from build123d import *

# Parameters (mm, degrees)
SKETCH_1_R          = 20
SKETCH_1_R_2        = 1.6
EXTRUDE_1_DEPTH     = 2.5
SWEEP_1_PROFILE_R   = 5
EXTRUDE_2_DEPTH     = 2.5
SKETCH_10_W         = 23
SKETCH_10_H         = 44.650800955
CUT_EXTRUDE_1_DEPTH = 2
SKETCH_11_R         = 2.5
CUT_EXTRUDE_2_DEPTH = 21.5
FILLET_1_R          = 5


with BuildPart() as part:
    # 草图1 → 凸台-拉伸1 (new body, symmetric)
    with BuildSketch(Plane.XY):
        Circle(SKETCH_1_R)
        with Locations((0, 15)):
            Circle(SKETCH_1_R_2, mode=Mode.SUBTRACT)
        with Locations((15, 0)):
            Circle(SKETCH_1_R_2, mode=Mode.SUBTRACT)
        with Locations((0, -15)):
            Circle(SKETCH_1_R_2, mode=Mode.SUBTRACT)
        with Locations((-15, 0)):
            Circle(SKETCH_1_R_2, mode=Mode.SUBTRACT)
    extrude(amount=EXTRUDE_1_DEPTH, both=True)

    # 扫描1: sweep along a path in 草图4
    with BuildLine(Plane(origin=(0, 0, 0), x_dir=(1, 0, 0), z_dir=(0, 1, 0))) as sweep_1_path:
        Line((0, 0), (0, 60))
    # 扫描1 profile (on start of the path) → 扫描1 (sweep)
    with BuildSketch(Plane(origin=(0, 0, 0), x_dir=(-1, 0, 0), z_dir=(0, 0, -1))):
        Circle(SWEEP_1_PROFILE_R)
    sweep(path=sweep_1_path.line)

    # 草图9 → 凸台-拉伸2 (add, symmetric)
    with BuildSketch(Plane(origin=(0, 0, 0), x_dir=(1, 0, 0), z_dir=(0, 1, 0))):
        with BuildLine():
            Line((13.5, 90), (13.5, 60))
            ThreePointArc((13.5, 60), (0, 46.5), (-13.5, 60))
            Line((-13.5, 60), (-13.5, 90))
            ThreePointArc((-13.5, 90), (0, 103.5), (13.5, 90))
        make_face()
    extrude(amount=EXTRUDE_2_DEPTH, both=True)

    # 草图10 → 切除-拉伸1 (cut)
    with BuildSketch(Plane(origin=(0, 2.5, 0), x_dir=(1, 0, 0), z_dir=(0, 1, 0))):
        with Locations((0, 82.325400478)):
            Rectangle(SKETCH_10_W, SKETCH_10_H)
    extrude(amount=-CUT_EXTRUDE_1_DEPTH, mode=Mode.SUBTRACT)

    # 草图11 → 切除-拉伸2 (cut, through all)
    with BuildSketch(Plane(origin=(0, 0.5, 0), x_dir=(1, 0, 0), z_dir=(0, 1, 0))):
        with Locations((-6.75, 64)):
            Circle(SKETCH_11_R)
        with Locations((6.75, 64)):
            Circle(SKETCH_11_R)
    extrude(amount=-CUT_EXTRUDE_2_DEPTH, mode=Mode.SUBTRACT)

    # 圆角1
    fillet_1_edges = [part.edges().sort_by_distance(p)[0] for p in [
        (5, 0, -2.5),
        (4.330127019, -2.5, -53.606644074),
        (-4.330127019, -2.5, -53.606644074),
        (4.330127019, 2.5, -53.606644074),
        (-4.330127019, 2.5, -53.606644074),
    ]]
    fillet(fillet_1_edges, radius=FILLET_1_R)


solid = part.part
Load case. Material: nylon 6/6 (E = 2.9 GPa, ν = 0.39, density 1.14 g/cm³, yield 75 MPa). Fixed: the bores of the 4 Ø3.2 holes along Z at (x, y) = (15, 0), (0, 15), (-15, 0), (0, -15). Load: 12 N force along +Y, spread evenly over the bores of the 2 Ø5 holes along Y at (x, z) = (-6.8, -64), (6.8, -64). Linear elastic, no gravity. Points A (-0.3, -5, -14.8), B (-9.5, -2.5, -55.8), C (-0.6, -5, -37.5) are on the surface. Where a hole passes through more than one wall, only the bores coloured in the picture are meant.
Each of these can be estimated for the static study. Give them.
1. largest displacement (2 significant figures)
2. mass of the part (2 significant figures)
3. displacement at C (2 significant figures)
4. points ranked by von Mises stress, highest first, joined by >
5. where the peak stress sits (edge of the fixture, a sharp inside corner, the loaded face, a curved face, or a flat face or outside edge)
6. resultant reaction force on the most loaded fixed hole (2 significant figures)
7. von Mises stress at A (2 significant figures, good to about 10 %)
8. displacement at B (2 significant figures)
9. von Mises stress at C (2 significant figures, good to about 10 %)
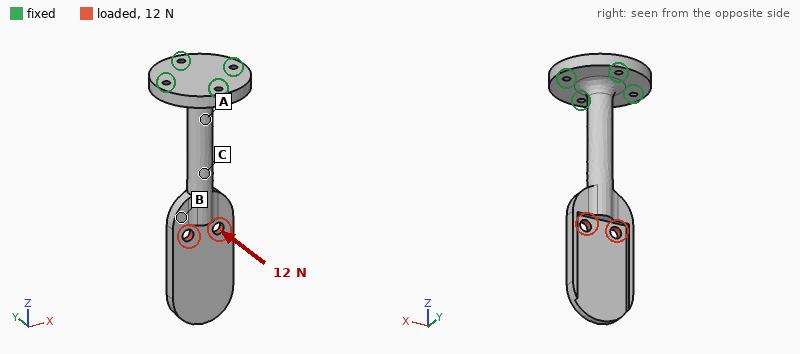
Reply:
1.3 mm
17 g
0.27 mm
A > C > B
a curved face
28 N
6.0 MPa
0.54 mm
3.2 MPa
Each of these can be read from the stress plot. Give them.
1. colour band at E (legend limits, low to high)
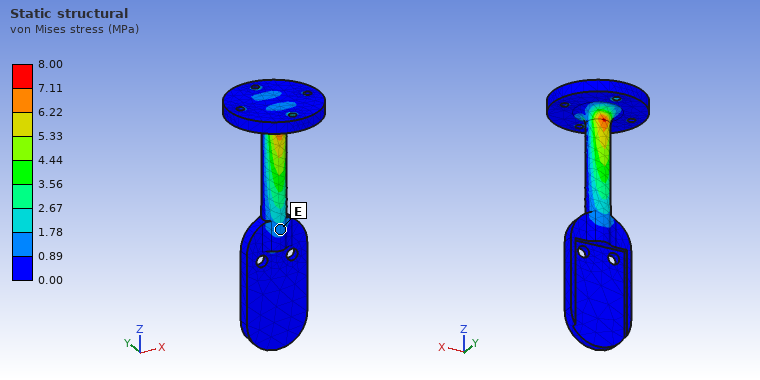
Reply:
0.89 to 1.78 MPa
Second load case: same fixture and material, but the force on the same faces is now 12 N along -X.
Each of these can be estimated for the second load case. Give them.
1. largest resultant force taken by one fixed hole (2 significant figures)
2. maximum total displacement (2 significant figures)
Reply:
28 N
1.3 mm
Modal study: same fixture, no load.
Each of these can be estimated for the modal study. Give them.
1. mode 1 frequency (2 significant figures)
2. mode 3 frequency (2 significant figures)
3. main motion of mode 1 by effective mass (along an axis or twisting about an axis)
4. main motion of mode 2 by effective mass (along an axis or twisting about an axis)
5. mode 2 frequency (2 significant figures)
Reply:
200 Hz
850 Hz
along Y
along X
220 Hz
